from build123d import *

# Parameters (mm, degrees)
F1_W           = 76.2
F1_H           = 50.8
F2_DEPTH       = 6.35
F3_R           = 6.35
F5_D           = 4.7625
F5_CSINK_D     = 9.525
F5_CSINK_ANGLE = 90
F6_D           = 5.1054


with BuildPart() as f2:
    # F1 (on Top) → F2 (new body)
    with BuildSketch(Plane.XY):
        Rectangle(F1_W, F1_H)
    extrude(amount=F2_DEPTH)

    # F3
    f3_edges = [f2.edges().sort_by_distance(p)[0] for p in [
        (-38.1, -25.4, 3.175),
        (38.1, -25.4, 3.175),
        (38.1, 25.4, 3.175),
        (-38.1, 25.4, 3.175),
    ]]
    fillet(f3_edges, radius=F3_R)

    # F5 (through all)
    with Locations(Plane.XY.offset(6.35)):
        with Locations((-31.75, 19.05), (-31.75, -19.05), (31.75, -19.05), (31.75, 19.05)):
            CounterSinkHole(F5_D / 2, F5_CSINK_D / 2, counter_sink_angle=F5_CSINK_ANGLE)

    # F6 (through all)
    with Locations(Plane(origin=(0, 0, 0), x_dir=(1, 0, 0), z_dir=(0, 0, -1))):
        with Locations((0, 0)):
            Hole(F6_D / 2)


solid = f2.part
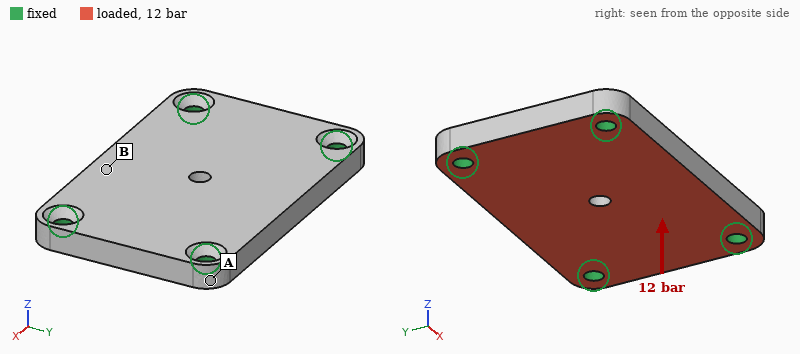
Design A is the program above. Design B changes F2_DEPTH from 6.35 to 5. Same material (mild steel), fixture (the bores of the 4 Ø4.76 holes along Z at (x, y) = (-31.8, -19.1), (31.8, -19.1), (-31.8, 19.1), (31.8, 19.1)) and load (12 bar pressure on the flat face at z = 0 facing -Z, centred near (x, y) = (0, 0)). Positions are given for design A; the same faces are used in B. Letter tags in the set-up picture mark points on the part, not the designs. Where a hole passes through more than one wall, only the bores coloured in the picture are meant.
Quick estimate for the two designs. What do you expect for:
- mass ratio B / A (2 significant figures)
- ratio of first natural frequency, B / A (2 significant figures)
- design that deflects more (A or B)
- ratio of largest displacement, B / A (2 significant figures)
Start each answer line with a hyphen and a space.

- 0.79
- 0.89
- B
- 1.6
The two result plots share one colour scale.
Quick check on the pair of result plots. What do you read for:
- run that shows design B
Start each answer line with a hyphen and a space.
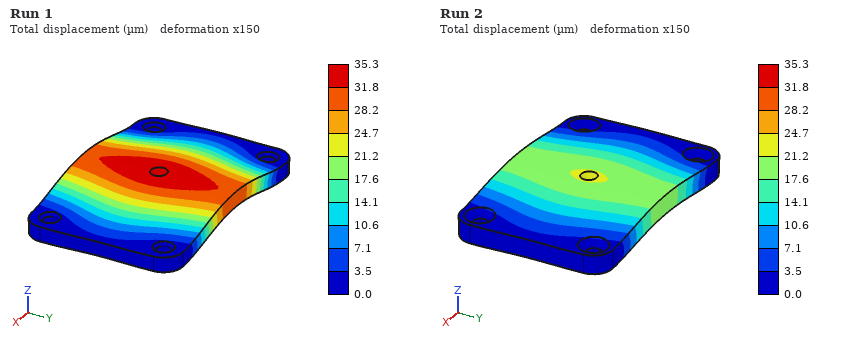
- Run 1
